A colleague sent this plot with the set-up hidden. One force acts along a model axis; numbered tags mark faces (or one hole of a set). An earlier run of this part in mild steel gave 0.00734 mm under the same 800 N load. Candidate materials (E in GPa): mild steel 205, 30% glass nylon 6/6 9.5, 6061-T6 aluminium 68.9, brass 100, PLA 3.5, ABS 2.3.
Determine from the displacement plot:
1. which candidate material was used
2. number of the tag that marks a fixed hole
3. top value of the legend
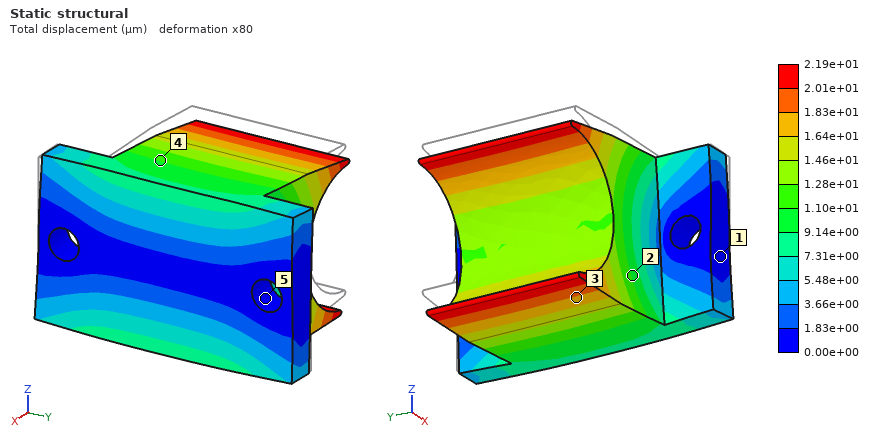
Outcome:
6061-T6 aluminium
5
2.19e+01 µm
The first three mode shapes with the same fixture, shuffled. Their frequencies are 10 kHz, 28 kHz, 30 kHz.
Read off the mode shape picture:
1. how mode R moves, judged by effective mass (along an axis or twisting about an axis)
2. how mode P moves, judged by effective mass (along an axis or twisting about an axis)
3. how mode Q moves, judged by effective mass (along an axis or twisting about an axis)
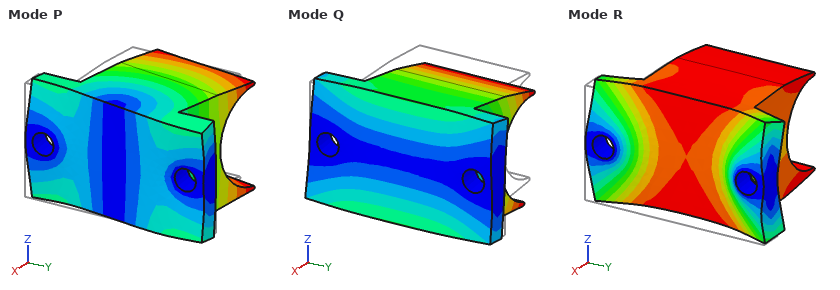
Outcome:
along X
along Y
along Z
